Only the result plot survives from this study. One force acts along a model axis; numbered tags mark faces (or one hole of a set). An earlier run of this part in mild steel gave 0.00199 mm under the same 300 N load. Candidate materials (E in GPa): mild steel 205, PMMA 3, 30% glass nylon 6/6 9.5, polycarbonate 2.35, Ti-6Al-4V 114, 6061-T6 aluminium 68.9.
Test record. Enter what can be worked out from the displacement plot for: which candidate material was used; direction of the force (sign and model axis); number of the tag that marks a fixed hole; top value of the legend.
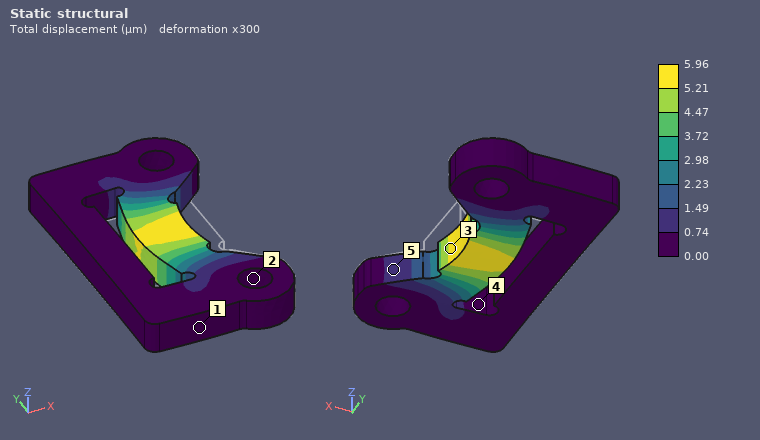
6061-T6 aluminium
-X
2
5.96 µm
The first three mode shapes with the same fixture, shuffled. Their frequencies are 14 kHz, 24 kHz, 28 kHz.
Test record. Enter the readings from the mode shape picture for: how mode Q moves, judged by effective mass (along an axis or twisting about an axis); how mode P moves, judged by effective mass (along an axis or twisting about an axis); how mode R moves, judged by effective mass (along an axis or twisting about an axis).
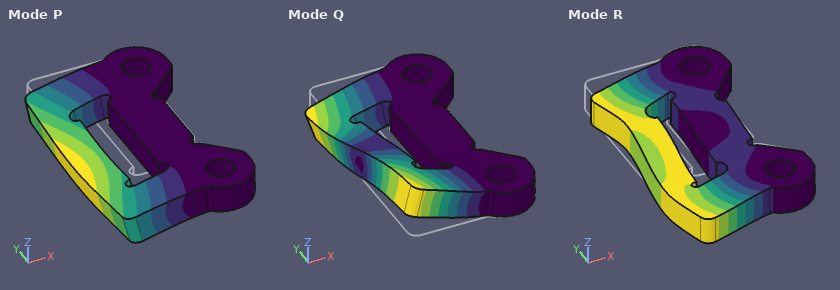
twisting about X
along Z
along Y
